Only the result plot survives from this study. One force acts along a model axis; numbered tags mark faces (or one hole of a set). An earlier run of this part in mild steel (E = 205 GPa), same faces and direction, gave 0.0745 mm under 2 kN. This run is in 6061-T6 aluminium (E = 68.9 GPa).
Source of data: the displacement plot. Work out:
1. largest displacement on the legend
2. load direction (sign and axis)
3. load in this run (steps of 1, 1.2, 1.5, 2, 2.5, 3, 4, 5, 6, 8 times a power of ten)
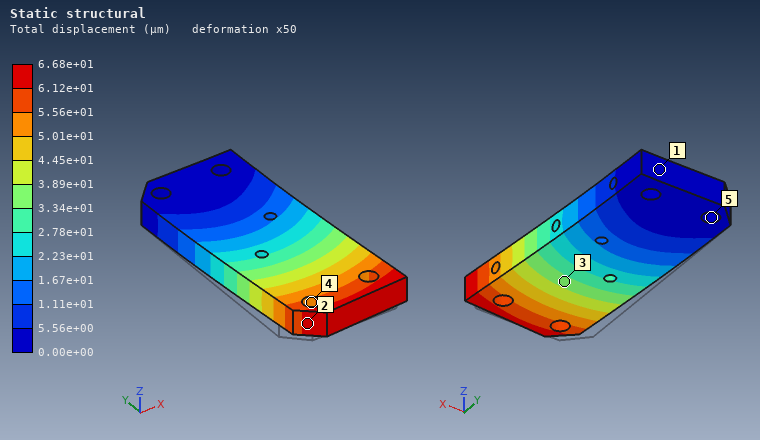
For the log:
6.68e+01 µm
+X
600 N
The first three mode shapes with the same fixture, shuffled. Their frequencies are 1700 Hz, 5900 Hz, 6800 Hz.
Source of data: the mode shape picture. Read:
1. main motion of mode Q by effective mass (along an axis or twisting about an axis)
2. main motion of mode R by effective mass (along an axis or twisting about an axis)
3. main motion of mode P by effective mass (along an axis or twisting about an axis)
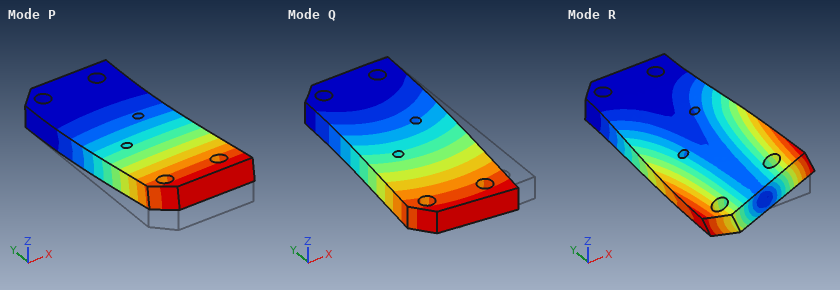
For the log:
along X
twisting about Y
along Z
